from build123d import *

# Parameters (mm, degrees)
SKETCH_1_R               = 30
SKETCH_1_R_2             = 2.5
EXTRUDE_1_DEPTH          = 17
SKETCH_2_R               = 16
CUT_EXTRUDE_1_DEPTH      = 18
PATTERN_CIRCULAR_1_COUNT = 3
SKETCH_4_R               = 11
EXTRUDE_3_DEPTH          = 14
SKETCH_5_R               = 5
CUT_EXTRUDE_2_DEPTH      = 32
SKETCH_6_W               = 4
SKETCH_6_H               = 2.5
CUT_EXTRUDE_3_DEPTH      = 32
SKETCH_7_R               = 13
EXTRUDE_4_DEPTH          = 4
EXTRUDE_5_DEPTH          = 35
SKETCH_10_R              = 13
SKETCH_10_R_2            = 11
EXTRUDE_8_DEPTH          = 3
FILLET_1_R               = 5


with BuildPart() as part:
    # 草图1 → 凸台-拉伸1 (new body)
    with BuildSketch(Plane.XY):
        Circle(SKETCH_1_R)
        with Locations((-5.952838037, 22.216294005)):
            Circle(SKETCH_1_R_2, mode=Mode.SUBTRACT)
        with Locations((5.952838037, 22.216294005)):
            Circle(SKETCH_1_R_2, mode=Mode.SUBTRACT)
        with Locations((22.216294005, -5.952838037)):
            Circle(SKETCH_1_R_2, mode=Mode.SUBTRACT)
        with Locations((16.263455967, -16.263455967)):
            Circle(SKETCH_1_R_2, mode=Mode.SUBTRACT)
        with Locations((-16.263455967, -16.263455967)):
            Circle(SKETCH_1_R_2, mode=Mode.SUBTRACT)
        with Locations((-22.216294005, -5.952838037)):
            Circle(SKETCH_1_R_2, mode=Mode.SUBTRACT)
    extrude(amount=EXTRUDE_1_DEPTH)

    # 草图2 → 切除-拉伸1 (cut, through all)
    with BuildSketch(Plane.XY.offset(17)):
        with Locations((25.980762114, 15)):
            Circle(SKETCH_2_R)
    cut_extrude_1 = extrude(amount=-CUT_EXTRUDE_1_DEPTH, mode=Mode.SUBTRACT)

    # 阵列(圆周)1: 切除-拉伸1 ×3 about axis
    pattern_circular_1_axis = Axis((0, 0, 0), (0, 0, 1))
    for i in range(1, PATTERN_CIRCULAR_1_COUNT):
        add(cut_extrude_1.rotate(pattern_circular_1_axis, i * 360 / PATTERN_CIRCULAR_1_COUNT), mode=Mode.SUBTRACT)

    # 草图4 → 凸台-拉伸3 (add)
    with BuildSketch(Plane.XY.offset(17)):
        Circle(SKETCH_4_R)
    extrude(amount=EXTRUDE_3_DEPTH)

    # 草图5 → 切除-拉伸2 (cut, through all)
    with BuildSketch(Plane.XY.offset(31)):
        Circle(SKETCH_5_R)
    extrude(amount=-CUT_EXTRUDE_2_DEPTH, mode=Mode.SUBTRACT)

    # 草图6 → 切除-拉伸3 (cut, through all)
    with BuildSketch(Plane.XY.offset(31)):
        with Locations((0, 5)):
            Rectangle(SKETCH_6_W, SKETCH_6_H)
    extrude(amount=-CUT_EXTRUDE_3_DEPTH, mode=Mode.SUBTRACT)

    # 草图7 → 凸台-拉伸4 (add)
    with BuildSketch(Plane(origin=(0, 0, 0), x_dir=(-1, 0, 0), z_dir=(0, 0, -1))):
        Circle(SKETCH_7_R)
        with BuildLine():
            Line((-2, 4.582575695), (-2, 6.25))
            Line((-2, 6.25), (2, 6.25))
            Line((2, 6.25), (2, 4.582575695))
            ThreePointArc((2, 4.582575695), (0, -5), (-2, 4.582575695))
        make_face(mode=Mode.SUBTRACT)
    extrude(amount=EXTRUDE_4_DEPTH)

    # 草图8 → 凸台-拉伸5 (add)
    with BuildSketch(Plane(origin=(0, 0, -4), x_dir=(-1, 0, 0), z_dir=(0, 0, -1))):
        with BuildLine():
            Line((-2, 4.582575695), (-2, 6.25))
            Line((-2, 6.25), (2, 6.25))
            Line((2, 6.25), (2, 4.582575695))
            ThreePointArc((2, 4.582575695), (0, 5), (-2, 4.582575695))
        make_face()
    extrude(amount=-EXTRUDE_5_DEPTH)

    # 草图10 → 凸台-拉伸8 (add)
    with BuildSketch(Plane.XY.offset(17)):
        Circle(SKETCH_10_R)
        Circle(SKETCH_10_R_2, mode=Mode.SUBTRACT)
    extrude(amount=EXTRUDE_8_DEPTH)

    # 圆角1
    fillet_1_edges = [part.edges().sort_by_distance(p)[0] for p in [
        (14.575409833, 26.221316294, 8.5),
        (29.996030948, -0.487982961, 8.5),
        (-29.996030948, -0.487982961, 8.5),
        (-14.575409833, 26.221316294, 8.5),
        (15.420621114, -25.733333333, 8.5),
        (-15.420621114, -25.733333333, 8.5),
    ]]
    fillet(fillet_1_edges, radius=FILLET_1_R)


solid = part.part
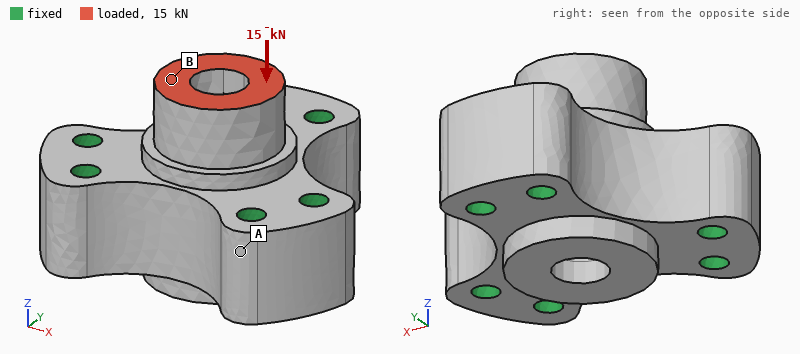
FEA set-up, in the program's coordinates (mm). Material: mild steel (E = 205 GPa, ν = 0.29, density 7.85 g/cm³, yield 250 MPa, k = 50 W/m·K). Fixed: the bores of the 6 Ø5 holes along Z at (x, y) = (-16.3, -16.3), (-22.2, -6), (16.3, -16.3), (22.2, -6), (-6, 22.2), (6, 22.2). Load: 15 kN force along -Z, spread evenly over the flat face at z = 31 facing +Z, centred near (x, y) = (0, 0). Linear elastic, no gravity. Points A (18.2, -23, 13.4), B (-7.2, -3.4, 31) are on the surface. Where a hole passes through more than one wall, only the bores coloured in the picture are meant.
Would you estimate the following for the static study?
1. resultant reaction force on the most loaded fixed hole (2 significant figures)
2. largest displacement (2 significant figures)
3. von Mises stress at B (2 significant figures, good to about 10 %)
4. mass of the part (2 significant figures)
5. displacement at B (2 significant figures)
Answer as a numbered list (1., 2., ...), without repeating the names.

1. 2.6 kN
2. 6.7 µm
3. 51 MPa
4. 250 g
5. 6.5 µm
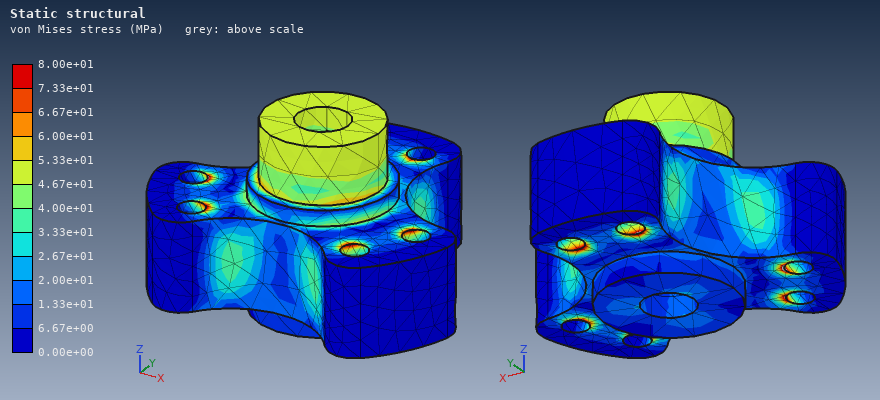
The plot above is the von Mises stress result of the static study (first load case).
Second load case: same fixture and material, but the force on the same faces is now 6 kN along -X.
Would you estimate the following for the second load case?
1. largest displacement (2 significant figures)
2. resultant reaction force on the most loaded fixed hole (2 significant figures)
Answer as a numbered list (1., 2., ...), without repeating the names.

1. 14 µm
2. 2.8 kN
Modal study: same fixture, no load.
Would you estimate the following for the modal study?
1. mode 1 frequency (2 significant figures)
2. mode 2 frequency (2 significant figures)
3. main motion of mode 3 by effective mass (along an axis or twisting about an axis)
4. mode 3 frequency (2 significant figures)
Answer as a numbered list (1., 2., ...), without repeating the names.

1. 29 kHz
2. 29 kHz
3. along Z
4. 32 kHz
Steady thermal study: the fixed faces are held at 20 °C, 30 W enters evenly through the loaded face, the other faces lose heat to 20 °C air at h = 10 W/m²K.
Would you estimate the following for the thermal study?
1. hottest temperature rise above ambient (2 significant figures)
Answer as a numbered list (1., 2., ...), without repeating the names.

1. 38 K
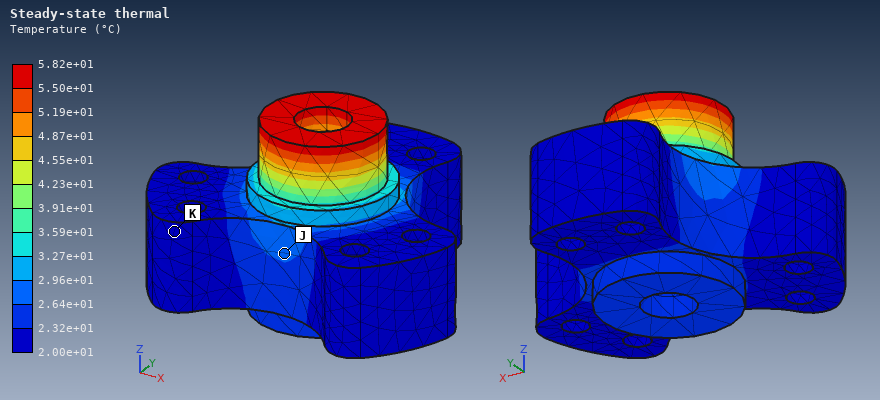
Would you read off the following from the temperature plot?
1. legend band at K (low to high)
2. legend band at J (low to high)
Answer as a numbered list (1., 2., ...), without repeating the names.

1. 2.00e+01 to 2.32e+01 °C
2. 2.64e+01 to 2.96e+01 °C
